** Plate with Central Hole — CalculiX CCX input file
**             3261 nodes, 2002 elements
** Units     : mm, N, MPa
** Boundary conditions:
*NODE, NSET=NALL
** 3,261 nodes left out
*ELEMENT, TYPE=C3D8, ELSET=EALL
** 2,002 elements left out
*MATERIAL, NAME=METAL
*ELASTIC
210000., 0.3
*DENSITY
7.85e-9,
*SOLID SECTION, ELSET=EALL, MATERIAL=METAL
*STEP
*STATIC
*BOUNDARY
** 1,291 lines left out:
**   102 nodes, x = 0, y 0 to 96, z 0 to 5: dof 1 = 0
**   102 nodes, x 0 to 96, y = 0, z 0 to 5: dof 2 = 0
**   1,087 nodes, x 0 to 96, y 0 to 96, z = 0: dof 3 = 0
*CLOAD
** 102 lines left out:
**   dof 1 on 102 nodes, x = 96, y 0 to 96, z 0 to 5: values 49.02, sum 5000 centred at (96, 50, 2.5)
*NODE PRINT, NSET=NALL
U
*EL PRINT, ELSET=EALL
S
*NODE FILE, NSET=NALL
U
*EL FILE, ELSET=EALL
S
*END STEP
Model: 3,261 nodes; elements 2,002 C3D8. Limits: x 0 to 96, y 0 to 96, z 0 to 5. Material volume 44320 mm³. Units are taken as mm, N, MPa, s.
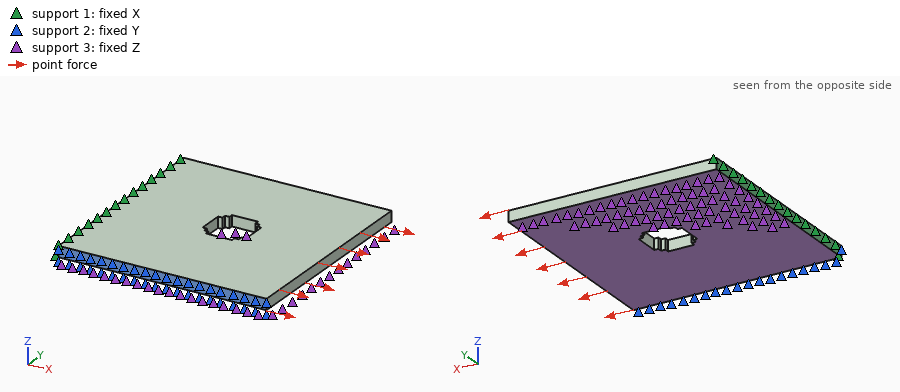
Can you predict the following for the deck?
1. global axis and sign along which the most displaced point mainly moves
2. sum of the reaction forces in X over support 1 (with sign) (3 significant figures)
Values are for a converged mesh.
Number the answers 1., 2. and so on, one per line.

1. +X
2. -5000 N
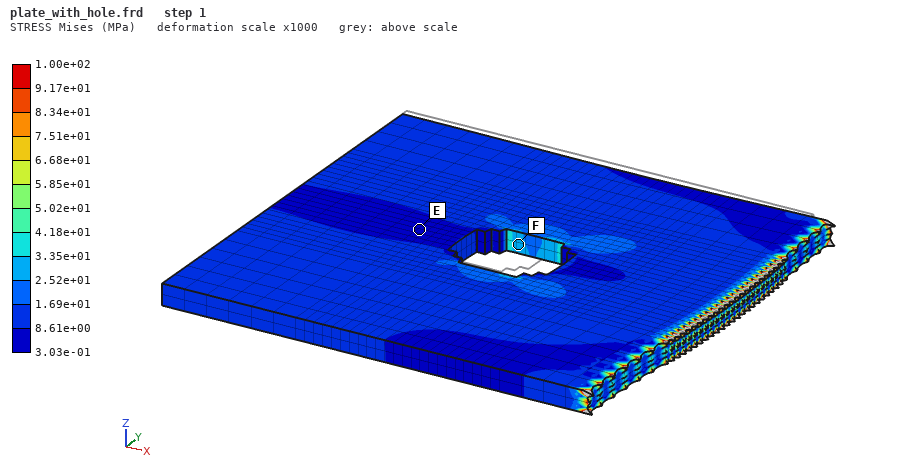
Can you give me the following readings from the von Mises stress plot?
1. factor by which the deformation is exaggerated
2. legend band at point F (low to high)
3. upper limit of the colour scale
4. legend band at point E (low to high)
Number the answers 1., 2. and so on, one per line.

1. 1000
2. 2.52e+01 to 3.35e+01 MPa
3. 1.00e+02 MPa
4. 3.03e-01 to 8.61e+00 MPa
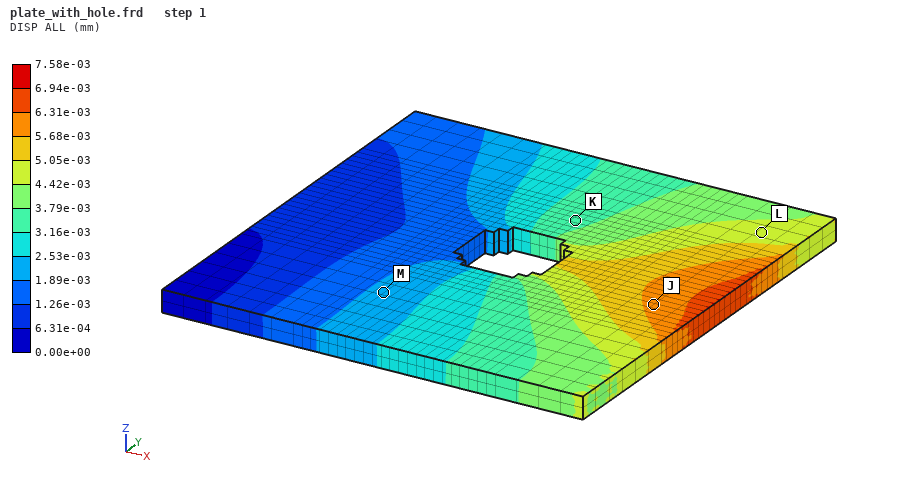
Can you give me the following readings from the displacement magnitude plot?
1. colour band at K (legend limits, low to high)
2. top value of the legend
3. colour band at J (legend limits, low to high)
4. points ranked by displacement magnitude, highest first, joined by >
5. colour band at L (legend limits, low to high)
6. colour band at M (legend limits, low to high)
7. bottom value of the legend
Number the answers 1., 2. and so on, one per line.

1. 3.16e-03 to 3.79e-03 mm
2. 7.58e-03 mm
3. 5.68e-03 to 6.31e-03 mm
4. J > L > K > M
5. 4.42e-03 to 5.05e-03 mm
6. 1.89e-03 to 2.53e-03 mm
7. 0.00e+00 mm
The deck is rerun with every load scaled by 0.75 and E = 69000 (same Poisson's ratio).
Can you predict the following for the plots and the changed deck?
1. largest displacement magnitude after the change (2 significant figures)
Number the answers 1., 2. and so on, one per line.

1. 0.017 mm
